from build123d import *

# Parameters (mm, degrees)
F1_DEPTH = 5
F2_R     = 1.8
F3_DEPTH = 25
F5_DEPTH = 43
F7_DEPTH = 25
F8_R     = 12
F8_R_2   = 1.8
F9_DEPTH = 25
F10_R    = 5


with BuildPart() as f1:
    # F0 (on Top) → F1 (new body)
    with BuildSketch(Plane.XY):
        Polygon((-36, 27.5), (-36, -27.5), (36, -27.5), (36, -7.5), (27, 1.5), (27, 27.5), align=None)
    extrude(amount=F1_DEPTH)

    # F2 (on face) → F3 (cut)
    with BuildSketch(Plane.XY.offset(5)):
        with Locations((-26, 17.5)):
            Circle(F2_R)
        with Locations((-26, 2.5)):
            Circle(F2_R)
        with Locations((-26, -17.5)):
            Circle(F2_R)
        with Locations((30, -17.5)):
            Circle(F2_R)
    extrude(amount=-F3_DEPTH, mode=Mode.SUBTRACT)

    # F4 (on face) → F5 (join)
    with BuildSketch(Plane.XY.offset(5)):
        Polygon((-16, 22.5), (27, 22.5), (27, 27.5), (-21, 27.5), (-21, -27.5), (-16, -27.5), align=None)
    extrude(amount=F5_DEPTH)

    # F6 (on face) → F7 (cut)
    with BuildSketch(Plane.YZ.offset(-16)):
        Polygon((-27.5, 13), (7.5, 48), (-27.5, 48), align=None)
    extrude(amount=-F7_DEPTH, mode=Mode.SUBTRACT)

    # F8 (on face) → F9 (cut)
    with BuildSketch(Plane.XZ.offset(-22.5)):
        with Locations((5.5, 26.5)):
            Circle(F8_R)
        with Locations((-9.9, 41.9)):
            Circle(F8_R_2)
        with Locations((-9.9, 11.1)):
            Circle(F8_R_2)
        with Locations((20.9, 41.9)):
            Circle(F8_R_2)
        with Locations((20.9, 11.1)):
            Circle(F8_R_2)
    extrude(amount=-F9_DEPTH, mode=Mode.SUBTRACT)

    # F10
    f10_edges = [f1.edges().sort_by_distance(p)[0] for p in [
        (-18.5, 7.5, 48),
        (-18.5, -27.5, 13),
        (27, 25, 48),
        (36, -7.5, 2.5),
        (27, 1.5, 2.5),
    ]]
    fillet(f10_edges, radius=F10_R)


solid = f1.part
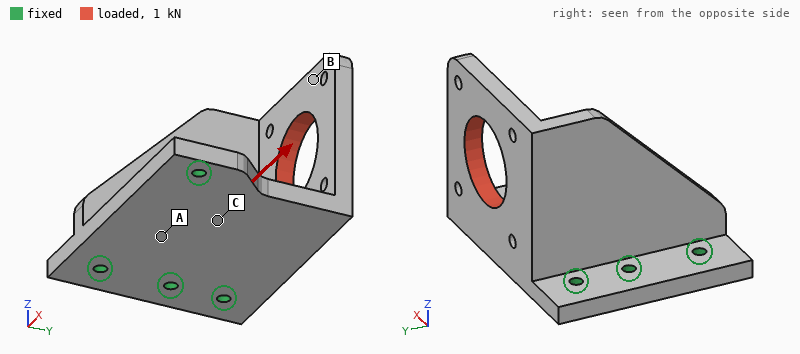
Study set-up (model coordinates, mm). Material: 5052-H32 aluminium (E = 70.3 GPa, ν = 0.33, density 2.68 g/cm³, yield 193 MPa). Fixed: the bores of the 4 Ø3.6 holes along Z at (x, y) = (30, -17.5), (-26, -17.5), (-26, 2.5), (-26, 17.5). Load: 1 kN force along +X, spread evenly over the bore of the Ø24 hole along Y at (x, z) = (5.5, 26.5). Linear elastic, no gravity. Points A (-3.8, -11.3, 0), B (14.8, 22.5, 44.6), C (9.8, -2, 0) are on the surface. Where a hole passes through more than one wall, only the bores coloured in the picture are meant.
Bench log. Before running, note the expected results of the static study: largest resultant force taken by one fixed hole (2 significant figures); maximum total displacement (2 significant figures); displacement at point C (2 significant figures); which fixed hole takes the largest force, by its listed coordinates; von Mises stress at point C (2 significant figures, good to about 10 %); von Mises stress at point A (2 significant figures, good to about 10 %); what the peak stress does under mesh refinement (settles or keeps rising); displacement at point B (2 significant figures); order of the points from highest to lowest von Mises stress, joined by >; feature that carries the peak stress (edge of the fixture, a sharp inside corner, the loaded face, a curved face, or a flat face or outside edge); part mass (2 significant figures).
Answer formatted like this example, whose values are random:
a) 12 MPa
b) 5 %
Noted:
a) 700 N
b) 0.27 mm
c) 0.040 mm
d) (-26, 17.5)
e) 26 MPa
f) 17 MPa
g) keeps rising
h) 0.23 mm
i) C > A > B
j) edge of the fixture
k) 90 g
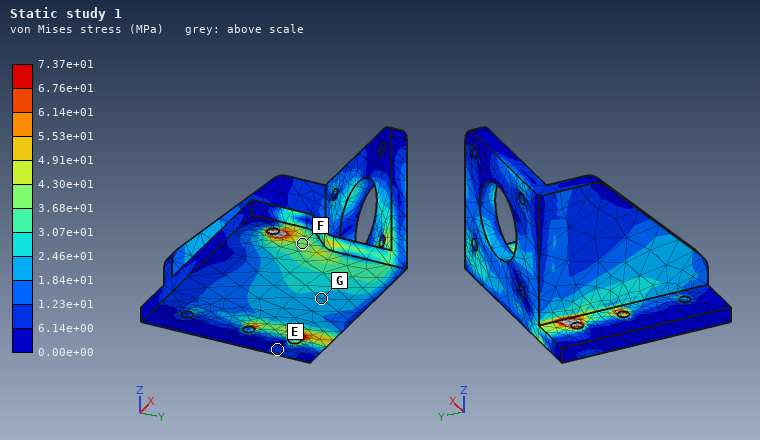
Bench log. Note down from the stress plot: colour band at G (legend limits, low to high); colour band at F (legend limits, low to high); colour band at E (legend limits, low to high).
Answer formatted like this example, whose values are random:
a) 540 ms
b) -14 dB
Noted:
a) 1.84e+01 to 2.46e+01 MPa
b) 3.68e+01 to 4.30e+01 MPa
c) 6.14e+00 to 1.23e+01 MPa
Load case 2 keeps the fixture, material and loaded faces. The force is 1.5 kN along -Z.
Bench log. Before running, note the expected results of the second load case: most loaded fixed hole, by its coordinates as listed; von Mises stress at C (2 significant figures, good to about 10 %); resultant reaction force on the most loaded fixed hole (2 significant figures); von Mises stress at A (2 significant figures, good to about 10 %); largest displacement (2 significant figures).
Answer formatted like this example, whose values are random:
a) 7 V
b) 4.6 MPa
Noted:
a) (-26, 17.5)
b) 46 MPa
c) 1.3 kN
d) 29 MPa
e) 0.47 mm
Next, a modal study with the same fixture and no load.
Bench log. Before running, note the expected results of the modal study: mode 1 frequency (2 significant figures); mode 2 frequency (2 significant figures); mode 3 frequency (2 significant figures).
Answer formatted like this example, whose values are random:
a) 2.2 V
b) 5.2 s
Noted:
a) 1700 Hz
b) 2900 Hz
c) 5700 Hz
